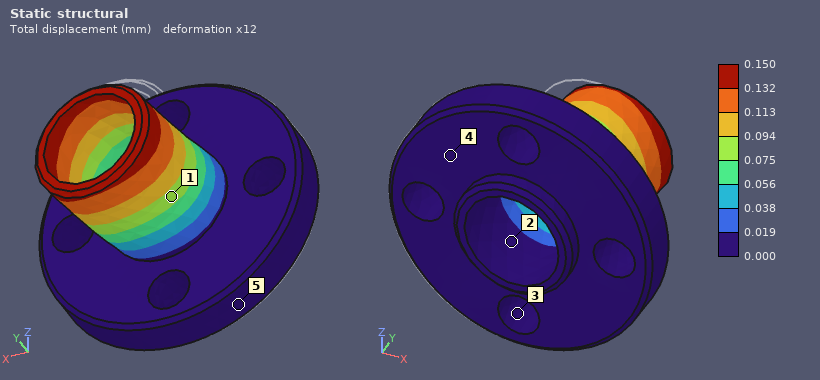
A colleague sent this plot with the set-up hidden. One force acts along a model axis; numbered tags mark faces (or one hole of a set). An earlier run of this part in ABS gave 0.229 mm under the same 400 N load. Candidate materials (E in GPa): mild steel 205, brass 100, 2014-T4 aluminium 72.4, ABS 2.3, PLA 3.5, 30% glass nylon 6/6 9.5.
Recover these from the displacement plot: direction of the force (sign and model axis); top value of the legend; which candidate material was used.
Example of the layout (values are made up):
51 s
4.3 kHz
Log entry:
+X
0.150 mm
PLA
